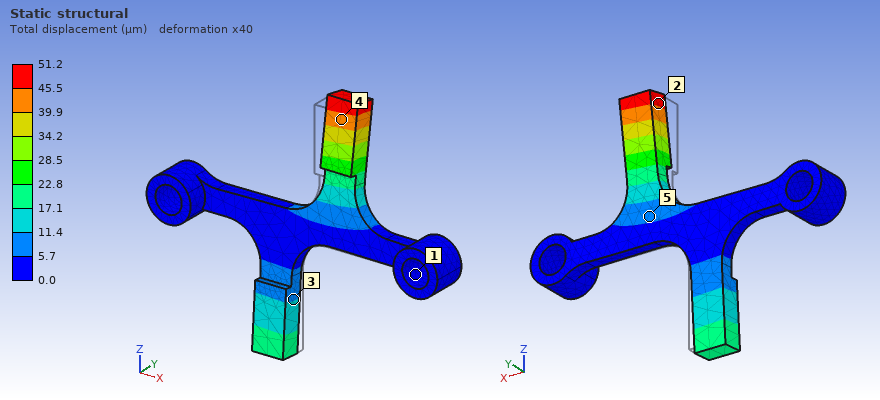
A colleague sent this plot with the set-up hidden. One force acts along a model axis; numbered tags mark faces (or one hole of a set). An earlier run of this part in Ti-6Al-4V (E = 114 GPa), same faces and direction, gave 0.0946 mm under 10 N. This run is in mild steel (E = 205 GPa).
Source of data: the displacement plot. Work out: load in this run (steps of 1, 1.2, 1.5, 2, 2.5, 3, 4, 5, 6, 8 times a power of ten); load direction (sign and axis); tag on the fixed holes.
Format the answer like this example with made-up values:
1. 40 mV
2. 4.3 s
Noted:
1. 10 N
2. +Y
3. 1
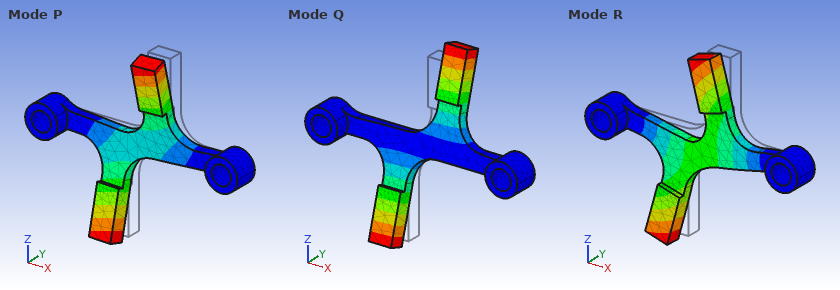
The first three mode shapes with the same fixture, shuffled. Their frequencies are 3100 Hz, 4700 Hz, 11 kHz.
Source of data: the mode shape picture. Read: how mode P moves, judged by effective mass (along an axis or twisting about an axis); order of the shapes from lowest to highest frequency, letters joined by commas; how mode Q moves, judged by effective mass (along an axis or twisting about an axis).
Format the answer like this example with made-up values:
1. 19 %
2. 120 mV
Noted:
1. along Y
2. Q, P, R
3. twisting about X
